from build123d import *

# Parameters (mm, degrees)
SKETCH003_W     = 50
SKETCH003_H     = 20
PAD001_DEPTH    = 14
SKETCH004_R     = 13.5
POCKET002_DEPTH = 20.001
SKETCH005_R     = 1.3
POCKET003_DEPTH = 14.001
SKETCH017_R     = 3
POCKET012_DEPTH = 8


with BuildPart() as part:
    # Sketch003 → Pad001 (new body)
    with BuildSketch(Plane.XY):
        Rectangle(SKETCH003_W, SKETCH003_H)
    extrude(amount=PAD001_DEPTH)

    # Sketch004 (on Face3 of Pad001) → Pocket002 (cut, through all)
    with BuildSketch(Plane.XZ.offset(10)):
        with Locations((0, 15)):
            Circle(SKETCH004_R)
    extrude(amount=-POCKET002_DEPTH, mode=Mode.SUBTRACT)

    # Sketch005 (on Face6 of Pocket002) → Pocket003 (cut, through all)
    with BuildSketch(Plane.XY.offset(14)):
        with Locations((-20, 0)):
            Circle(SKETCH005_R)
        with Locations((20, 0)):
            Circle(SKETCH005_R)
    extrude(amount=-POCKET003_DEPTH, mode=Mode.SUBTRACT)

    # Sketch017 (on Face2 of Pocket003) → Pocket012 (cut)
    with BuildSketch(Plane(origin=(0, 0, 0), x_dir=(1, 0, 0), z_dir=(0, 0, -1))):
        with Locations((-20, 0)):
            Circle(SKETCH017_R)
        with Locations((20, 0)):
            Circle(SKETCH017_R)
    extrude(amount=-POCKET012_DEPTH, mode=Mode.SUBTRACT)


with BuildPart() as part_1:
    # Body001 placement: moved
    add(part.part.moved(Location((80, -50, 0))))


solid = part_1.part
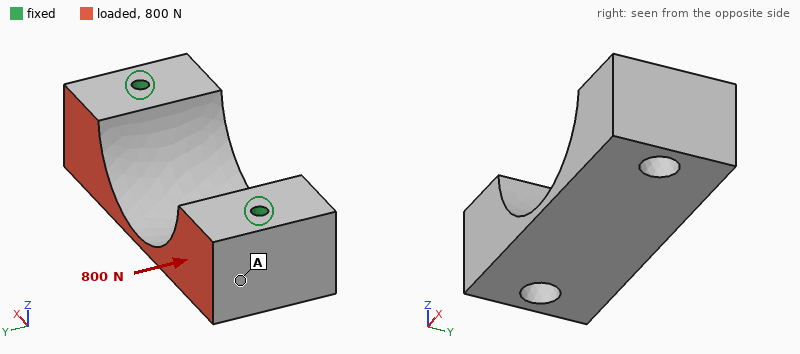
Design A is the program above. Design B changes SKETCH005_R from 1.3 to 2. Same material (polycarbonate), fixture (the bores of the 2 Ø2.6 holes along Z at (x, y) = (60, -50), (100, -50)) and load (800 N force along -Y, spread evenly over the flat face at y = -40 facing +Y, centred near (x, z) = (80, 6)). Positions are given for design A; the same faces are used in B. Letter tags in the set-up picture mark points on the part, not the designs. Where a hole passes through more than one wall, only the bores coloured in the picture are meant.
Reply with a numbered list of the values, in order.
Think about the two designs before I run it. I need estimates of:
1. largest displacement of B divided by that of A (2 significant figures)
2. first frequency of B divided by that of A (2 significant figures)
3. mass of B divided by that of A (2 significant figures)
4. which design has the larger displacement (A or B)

1. 0.67
2. 1.3
3. 0.99
4. A
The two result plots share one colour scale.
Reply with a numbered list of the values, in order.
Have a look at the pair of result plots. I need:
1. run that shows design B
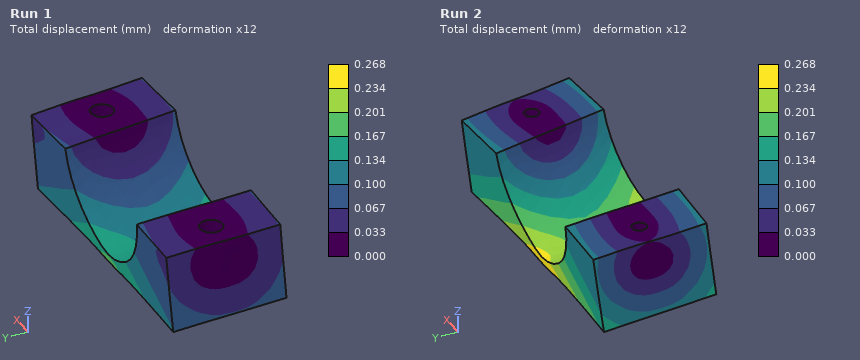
1. Run 1
